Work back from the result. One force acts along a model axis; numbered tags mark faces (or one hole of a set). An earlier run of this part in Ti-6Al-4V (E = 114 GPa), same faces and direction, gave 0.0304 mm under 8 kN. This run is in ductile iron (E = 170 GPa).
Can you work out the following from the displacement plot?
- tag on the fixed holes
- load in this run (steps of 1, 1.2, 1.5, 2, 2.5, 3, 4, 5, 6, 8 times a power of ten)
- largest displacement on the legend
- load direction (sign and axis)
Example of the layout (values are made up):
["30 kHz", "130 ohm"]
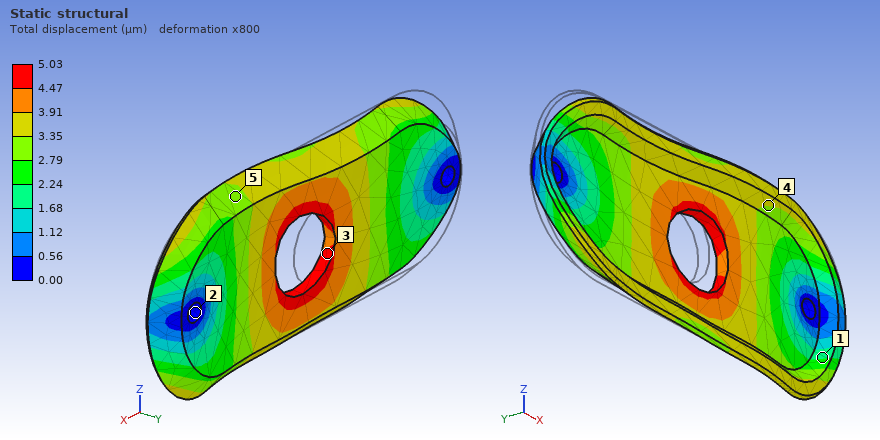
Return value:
["2", "2 kN", "5.03 µm", "+X"]
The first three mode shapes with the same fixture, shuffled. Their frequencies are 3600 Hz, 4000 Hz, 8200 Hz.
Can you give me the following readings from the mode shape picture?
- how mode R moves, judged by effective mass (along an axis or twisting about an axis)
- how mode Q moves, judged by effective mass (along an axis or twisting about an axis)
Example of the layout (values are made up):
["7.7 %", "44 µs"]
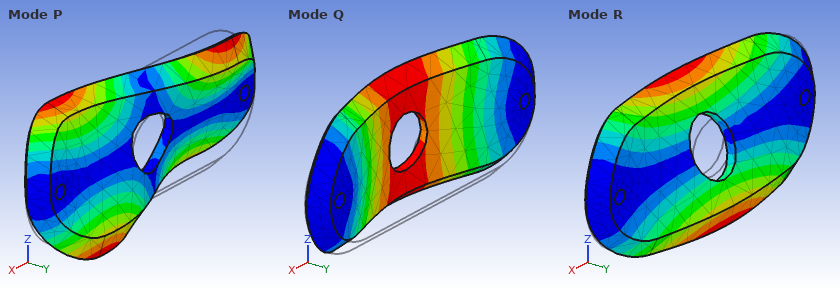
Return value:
["twisting about X", "along Y"]
